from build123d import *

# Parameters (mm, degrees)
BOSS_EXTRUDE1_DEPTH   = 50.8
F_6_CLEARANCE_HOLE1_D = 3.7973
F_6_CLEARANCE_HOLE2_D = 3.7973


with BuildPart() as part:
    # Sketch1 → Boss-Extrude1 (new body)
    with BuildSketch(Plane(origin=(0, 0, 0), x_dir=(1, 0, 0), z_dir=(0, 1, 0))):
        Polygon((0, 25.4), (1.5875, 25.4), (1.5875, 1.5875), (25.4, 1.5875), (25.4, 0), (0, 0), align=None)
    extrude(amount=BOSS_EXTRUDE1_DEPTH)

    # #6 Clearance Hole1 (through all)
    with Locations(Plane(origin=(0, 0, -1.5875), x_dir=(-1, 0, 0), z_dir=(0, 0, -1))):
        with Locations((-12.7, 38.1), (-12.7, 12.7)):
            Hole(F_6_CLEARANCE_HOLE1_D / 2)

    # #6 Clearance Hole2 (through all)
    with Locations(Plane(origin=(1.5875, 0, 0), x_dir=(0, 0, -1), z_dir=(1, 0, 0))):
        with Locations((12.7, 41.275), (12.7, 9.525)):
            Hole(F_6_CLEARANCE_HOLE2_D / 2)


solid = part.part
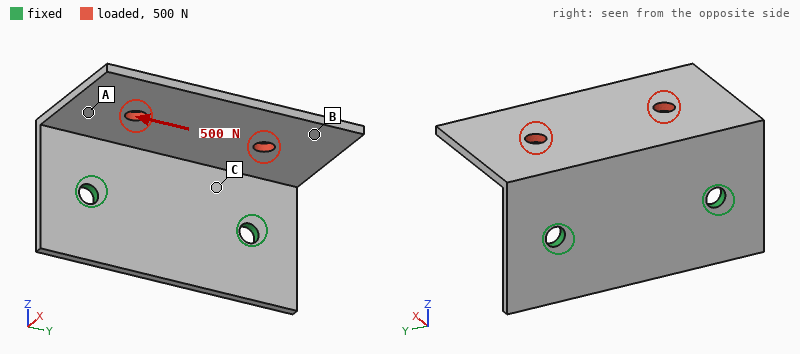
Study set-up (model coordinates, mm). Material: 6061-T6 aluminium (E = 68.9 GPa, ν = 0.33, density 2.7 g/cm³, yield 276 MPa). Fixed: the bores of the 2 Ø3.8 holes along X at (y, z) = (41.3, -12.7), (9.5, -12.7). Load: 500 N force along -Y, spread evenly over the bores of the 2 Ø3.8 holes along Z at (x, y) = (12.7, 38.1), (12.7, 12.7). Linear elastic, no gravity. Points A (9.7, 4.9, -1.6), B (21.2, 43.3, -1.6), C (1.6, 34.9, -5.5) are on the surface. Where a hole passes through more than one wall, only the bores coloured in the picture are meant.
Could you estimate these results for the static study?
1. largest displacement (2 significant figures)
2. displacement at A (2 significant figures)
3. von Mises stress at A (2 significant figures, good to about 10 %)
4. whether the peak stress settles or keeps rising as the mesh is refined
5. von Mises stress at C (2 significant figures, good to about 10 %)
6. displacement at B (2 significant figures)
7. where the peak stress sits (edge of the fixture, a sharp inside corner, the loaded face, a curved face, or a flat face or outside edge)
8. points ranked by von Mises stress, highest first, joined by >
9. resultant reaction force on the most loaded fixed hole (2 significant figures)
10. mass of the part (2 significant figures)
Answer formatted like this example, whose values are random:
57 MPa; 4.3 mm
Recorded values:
0.32 mm; 0.17 mm; 40 MPa; keeps rising; 77 MPa; 0.23 mm; edge of the fixture; C > A > B; 350 N; 11 g
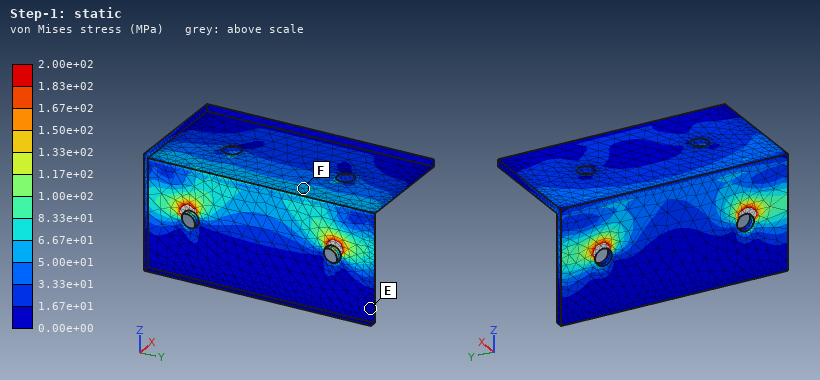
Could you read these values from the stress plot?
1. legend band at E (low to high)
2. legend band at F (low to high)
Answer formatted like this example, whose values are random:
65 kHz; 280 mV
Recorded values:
0.00e+00 to 1.67e+01 MPa; 5.00e+01 to 6.67e+01 MPa
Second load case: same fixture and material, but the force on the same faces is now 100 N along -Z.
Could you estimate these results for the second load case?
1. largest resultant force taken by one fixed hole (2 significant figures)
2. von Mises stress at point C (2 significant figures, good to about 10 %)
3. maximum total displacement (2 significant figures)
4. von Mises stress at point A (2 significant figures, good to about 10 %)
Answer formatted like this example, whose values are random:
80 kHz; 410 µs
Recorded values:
51 N; 52 MPa; 0.40 mm; 14 MPa
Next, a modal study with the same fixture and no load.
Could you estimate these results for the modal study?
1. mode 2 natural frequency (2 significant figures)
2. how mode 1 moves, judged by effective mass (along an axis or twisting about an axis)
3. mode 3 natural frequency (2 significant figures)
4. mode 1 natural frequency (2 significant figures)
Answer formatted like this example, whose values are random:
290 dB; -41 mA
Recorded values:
2300 Hz; along Z; 3900 Hz; 1200 Hz
